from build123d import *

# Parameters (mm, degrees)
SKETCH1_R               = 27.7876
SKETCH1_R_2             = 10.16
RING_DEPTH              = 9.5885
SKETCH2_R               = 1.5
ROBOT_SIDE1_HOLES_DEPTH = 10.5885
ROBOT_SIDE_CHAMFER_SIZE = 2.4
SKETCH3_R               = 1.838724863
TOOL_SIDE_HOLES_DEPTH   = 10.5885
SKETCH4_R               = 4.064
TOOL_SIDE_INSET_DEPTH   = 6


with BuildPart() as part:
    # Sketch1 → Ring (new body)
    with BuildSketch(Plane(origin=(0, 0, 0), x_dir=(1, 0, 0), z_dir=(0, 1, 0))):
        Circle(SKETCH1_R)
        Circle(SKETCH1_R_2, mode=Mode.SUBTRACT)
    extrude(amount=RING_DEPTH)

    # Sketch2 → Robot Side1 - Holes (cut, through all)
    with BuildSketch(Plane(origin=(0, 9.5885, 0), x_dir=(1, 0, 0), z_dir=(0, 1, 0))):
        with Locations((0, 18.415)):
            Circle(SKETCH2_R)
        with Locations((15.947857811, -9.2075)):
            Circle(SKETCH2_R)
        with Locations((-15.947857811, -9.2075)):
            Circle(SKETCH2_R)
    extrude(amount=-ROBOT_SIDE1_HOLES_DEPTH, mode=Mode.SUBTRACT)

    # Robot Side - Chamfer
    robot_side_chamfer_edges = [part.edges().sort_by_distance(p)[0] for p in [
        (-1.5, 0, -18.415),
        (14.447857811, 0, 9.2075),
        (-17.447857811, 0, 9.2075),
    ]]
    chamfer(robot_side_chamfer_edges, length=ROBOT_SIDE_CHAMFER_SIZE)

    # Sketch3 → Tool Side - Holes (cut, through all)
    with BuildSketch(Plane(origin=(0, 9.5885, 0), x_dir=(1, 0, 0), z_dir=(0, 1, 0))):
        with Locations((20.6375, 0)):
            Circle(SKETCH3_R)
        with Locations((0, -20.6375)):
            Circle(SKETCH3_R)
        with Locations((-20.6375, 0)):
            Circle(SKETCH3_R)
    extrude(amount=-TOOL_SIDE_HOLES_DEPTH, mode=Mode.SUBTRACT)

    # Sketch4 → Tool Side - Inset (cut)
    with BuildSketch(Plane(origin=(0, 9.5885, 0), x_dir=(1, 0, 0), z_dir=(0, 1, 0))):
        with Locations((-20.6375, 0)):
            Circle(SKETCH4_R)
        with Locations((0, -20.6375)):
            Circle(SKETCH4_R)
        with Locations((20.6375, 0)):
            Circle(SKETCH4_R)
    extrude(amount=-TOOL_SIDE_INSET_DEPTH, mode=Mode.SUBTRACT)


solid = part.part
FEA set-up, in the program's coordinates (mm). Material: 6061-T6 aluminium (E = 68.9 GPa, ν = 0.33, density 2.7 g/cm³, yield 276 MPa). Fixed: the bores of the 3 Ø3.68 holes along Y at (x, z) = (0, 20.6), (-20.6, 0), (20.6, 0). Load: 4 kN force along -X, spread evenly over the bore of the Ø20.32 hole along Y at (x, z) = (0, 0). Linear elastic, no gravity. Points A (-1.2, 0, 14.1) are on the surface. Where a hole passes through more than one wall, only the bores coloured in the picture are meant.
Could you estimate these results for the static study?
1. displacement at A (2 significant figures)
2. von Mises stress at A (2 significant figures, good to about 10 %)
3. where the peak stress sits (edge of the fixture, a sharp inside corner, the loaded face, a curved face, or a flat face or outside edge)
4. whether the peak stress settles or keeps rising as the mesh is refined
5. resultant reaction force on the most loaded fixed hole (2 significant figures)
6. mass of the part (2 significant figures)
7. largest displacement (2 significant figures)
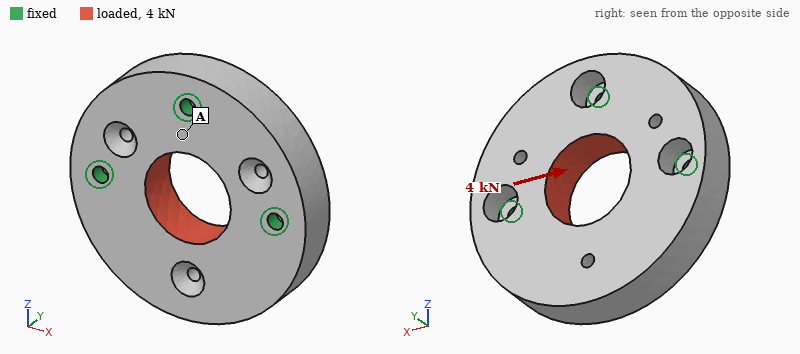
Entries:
2.3 µm
11 MPa
edge of the fixture
keeps rising
1.6 kN
51 g
7.4 µm
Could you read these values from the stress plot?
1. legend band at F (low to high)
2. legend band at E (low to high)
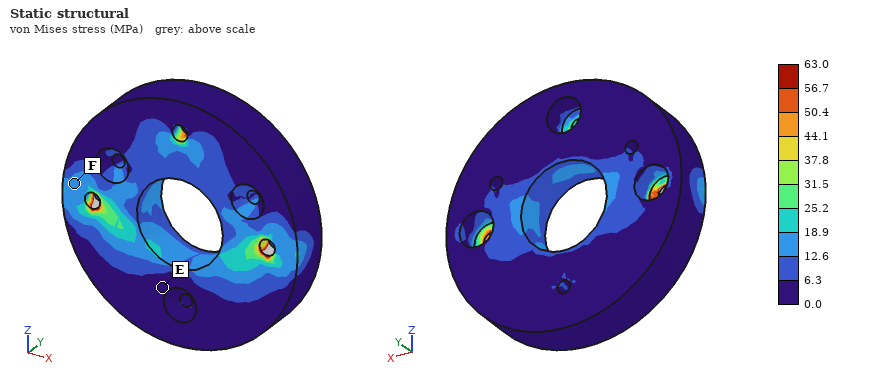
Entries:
12.6 to 18.9 MPa
0.0 to 6.3 MPa
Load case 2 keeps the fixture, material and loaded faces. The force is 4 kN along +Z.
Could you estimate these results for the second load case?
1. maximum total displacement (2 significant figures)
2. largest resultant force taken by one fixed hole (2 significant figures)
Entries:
23 µm
1.4 kN
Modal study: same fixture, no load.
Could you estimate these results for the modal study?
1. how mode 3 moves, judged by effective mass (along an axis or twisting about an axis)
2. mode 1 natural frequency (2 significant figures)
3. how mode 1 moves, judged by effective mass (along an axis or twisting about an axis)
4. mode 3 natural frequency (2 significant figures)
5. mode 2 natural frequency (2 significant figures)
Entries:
along X
5600 Hz
along Y
18 kHz
14 kHz
